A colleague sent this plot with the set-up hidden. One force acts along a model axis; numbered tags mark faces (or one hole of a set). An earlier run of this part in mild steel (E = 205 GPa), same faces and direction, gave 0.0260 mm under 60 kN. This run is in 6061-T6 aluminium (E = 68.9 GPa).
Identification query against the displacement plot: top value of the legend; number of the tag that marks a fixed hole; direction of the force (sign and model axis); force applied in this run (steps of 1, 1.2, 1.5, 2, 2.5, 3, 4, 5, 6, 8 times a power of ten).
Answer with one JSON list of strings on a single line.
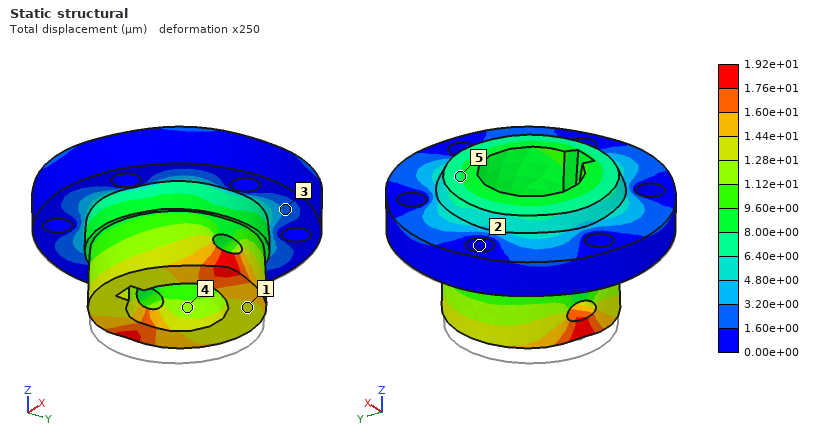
["1.92e+01 µm", "2", "+Z", "15 kN"]
